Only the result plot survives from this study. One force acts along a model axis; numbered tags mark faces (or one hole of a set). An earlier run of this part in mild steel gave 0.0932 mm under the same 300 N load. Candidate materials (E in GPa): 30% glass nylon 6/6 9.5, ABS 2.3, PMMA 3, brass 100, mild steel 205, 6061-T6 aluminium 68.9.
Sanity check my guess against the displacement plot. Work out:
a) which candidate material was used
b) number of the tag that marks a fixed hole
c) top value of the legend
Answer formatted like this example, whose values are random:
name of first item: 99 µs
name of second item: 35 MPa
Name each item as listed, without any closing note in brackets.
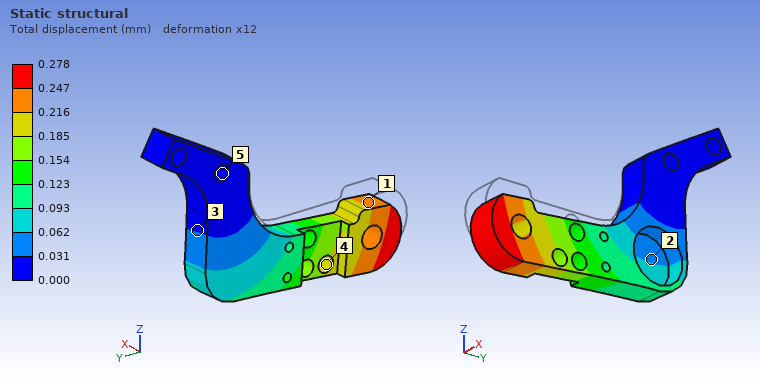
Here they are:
which candidate material was used: 6061-T6 aluminium
number of the tag that marks a fixed hole: 5
top value of the legend: 0.278 mm
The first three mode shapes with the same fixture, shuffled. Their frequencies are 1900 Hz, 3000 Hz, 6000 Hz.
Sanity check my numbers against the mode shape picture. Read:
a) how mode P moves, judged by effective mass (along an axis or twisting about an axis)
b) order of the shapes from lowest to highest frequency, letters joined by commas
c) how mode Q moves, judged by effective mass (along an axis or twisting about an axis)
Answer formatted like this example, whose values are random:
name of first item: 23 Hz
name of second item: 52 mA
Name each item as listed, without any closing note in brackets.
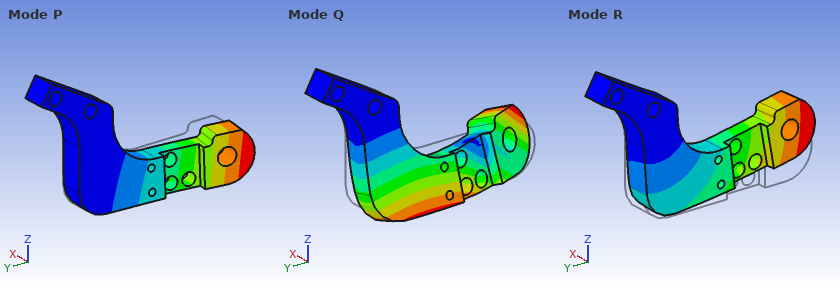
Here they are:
how mode P moves, judged by effective mass: along X
order of the shapes from lowest to highest frequency, letters joined by commas: P, R, Q
how mode Q moves, judged by effective mass: along X
